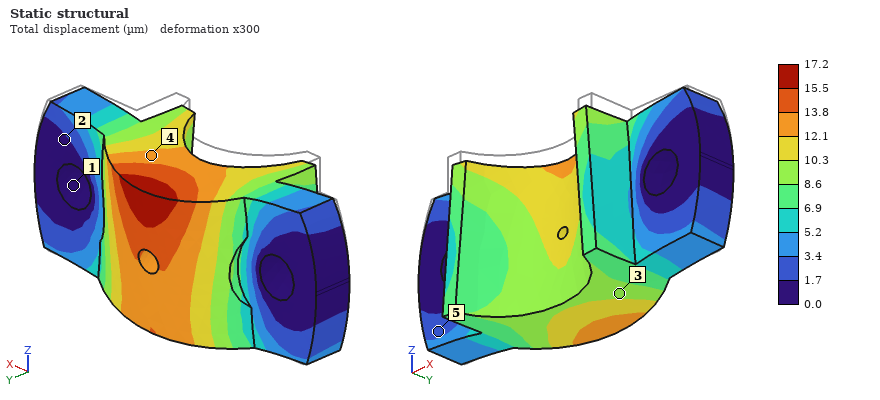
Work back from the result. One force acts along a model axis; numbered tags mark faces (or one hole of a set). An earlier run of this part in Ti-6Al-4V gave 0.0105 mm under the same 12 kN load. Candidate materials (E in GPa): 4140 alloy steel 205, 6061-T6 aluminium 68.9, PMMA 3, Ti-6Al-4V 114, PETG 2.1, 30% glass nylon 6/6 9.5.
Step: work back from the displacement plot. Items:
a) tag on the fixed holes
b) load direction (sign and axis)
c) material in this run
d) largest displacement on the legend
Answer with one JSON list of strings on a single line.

["1", "-Z", "6061-T6 aluminium", "17.2 µm"]
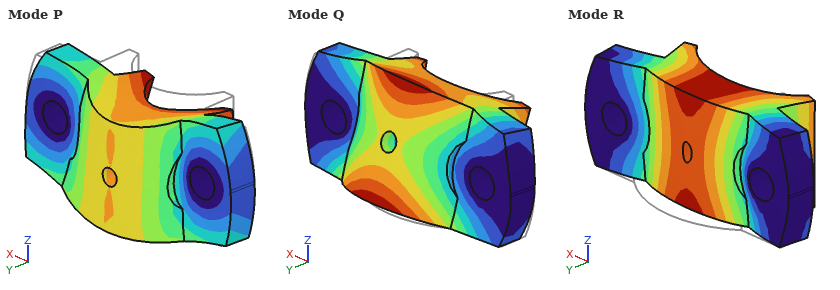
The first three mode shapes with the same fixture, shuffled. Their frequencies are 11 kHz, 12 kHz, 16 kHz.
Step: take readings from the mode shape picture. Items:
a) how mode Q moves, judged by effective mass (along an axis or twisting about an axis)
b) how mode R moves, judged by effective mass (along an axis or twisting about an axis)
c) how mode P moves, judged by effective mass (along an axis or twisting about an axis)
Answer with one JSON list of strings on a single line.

["twisting about X", "along Y", "along Z"]
